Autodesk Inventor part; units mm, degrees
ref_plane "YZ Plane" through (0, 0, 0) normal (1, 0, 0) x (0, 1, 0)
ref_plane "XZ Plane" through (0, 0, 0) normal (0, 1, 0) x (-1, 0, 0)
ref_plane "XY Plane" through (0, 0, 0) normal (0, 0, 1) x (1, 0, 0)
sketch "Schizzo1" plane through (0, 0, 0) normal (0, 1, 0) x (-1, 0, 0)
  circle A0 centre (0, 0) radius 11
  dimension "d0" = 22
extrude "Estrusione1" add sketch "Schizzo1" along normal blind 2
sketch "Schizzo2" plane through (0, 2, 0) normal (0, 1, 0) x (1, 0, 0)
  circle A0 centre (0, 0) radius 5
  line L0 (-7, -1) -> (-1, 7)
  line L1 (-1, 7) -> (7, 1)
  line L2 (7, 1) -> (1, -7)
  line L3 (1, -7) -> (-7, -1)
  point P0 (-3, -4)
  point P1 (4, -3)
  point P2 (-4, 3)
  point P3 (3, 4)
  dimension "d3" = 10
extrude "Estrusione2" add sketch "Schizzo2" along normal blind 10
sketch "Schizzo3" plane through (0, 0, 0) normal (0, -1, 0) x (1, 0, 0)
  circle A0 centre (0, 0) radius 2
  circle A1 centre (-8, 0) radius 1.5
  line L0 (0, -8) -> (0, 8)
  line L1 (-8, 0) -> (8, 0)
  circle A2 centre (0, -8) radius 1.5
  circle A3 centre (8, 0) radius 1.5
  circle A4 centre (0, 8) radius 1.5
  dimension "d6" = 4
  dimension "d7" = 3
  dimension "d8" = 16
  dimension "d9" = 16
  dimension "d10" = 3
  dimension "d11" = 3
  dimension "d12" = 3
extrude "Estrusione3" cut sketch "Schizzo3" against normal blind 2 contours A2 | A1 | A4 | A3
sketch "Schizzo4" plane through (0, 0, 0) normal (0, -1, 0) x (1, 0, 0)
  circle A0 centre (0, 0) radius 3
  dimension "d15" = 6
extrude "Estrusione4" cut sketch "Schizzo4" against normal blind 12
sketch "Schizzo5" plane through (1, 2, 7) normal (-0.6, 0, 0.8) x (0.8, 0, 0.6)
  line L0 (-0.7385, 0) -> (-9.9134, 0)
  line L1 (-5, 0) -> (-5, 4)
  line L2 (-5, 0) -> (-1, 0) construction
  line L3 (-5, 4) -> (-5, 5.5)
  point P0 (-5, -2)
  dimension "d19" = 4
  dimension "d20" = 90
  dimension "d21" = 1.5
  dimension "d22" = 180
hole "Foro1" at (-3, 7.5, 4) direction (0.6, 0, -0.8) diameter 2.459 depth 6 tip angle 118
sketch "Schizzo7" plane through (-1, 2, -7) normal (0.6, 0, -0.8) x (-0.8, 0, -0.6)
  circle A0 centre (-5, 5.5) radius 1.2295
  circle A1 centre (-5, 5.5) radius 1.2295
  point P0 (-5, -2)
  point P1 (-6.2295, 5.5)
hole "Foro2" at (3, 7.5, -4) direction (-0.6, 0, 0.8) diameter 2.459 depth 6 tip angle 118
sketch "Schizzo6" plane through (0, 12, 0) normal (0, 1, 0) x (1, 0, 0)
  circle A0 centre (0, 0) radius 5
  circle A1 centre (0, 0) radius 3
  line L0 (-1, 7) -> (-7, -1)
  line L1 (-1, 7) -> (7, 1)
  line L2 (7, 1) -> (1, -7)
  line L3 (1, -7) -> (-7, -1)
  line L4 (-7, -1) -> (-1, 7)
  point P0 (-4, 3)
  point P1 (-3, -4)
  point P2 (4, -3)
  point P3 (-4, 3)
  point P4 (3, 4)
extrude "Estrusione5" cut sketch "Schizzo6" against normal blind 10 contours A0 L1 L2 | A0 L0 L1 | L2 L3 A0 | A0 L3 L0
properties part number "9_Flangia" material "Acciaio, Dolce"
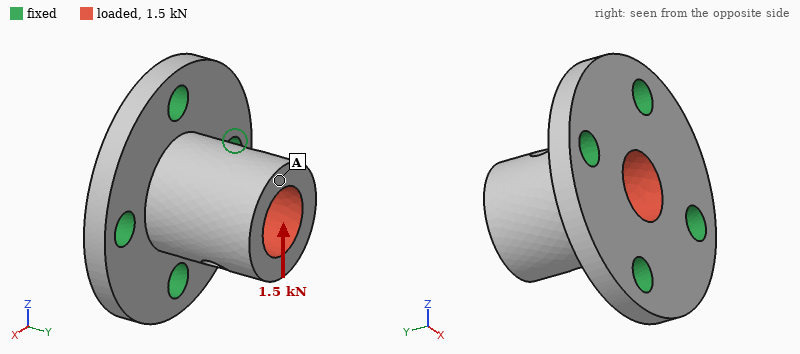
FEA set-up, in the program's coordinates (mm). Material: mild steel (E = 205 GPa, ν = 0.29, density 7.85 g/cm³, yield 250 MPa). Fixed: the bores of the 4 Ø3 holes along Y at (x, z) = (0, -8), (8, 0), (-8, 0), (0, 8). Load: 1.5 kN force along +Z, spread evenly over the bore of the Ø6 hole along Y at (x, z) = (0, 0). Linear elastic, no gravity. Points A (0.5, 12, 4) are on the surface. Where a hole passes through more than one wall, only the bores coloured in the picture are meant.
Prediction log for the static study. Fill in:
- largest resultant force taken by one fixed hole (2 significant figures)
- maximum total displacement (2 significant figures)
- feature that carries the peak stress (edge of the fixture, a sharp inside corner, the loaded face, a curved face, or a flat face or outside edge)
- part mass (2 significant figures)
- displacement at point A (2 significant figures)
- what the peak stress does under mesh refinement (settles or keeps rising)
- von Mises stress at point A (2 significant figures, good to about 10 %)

750 N
12 µm
edge of the fixture
8.9 g
12 µm
keeps rising
25 MPa
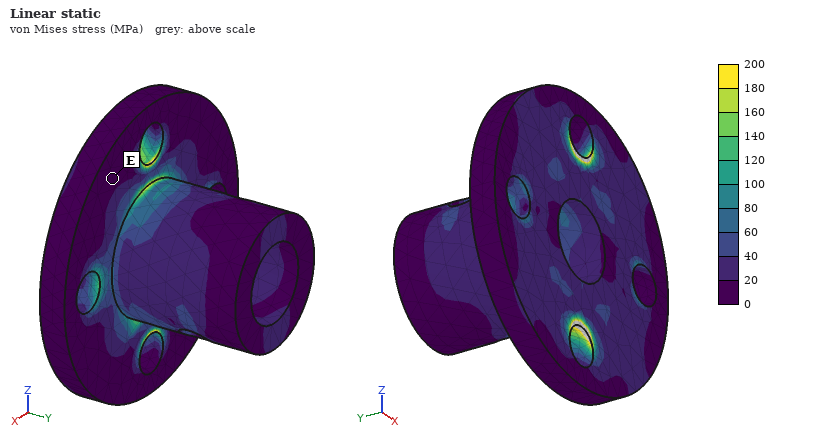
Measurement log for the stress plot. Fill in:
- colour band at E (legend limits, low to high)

0 to 20 MPa
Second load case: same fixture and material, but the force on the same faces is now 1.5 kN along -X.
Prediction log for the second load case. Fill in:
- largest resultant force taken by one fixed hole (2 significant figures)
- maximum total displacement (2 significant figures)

750 N
12 µm
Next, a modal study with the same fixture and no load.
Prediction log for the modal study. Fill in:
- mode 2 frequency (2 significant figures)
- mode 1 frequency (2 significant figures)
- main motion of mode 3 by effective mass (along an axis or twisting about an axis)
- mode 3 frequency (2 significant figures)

31 kHz
30 kHz
along Y
54 kHz
